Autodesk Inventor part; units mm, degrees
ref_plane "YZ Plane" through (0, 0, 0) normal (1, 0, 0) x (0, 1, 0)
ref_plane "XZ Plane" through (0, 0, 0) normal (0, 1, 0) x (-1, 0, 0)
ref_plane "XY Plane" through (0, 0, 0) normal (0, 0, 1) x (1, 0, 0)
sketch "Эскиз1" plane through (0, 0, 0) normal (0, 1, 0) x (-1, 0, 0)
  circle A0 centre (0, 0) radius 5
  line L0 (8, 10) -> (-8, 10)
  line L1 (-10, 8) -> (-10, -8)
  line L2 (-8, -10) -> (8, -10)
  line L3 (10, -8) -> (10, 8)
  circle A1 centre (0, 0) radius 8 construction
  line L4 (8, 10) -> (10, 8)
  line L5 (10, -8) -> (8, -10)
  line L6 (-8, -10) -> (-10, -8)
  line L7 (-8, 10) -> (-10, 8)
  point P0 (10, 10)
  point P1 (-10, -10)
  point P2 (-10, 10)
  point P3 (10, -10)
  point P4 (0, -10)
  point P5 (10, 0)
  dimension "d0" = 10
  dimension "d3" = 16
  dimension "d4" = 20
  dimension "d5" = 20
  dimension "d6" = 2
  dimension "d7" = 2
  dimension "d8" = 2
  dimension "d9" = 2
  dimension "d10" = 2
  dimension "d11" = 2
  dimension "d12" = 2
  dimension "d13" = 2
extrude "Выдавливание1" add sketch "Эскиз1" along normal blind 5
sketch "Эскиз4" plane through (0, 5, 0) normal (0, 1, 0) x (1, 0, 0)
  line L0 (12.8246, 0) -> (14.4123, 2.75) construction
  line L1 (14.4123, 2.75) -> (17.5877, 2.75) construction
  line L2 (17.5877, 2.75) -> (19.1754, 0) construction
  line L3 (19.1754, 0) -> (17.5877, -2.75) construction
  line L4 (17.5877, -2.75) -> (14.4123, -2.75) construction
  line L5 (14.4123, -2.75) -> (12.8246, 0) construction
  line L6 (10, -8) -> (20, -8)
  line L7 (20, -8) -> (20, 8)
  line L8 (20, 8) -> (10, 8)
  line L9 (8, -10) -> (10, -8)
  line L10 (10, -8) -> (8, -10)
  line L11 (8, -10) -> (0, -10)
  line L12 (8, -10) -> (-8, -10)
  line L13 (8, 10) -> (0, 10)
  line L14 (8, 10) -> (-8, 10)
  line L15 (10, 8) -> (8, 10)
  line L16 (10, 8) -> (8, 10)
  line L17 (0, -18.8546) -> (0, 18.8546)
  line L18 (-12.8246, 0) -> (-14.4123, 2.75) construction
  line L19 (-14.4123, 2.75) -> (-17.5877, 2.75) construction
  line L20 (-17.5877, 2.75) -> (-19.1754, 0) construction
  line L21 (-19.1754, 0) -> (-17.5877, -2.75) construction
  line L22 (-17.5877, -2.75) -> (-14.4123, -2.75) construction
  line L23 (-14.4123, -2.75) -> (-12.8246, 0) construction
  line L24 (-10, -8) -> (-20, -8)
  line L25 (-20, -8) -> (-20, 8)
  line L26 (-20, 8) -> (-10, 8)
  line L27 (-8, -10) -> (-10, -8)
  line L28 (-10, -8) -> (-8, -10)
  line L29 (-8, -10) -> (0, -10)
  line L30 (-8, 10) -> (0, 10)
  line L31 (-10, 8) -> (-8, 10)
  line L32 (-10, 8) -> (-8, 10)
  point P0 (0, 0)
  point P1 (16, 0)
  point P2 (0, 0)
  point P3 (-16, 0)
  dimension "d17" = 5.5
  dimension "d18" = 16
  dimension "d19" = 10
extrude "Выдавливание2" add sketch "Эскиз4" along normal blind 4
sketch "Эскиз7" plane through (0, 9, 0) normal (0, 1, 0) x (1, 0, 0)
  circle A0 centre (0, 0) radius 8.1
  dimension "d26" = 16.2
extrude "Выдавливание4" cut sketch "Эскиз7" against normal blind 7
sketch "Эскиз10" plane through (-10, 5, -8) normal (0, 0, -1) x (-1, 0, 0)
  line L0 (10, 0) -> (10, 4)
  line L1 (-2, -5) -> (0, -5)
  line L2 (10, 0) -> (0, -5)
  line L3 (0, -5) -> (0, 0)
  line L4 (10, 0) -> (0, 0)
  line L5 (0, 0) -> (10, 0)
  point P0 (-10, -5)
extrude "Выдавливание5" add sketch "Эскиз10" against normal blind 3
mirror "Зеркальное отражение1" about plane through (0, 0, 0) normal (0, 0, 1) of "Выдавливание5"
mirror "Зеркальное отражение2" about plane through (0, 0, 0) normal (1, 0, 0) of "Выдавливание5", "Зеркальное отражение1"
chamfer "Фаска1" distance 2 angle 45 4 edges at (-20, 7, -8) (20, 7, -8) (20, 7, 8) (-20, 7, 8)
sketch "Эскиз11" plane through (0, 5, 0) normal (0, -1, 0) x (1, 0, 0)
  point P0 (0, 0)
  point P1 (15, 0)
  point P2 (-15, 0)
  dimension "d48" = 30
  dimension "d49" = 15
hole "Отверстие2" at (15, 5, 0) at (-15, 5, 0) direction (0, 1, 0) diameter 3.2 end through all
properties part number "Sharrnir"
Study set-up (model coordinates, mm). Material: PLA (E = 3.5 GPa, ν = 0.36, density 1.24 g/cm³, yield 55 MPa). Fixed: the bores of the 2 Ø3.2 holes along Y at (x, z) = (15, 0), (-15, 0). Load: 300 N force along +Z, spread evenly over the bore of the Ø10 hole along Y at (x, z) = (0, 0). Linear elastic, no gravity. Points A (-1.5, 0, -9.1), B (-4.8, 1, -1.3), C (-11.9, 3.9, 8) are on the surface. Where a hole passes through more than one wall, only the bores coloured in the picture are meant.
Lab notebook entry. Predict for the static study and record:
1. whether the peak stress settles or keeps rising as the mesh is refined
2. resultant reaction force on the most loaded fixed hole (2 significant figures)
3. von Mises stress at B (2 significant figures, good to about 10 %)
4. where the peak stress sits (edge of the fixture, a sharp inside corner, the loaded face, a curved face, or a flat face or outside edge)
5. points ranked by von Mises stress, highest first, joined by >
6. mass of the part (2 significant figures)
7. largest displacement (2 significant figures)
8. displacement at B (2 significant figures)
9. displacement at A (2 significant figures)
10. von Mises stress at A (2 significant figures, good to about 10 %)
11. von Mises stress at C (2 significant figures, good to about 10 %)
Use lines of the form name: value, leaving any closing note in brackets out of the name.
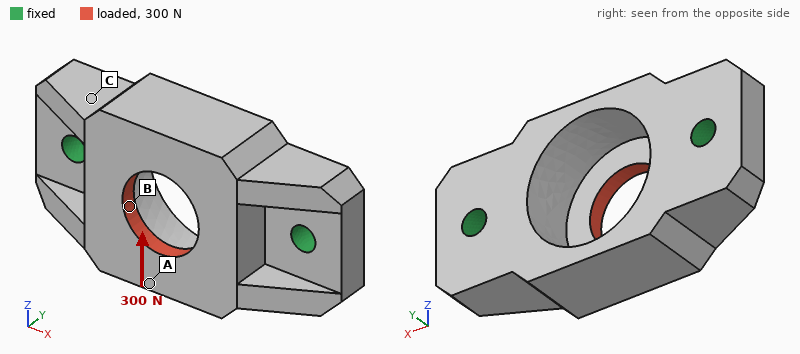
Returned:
whether the peak stress settles or keeps rising as the mesh is refined: keeps rising
resultant reaction force on the most loaded fixed hole: 150 N
von Mises stress at B: 10.0 MPa
where the peak stress sits: edge of the fixture
points ranked by von Mises stress, highest first, joined by >: B > C > A
mass of the part: 4.2 g
largest displacement: 0.17 mm
displacement at B: 0.100 mm
displacement at A: 0.16 mm
von Mises stress at A: 3.4 MPa
von Mises stress at C: 6.2 MPa
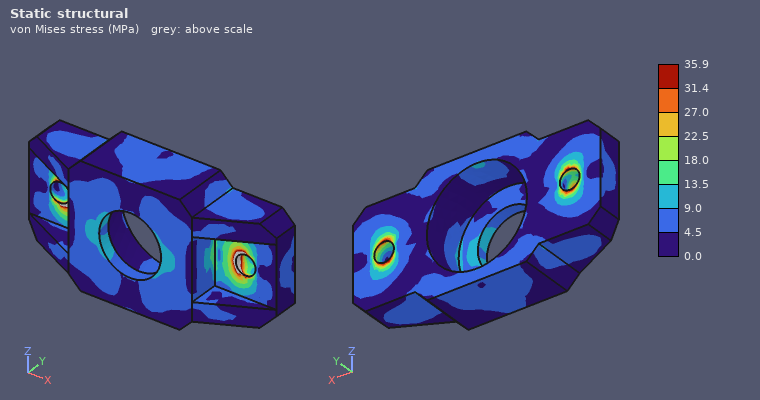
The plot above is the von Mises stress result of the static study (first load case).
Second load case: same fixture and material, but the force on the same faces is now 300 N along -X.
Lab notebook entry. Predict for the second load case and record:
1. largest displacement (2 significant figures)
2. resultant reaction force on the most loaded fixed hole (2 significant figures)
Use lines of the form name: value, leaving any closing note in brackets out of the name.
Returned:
largest displacement: 41 µm
resultant reaction force on the most loaded fixed hole: 160 N
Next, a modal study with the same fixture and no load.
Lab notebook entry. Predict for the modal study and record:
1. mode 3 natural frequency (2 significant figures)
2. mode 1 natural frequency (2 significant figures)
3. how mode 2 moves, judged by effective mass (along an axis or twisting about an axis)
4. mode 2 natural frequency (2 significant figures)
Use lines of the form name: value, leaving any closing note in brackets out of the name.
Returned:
mode 3 natural frequency: 10 kHz
mode 1 natural frequency: 4800 Hz
how mode 2 moves, judged by effective mass: along Y
mode 2 natural frequency: 7900 Hz
